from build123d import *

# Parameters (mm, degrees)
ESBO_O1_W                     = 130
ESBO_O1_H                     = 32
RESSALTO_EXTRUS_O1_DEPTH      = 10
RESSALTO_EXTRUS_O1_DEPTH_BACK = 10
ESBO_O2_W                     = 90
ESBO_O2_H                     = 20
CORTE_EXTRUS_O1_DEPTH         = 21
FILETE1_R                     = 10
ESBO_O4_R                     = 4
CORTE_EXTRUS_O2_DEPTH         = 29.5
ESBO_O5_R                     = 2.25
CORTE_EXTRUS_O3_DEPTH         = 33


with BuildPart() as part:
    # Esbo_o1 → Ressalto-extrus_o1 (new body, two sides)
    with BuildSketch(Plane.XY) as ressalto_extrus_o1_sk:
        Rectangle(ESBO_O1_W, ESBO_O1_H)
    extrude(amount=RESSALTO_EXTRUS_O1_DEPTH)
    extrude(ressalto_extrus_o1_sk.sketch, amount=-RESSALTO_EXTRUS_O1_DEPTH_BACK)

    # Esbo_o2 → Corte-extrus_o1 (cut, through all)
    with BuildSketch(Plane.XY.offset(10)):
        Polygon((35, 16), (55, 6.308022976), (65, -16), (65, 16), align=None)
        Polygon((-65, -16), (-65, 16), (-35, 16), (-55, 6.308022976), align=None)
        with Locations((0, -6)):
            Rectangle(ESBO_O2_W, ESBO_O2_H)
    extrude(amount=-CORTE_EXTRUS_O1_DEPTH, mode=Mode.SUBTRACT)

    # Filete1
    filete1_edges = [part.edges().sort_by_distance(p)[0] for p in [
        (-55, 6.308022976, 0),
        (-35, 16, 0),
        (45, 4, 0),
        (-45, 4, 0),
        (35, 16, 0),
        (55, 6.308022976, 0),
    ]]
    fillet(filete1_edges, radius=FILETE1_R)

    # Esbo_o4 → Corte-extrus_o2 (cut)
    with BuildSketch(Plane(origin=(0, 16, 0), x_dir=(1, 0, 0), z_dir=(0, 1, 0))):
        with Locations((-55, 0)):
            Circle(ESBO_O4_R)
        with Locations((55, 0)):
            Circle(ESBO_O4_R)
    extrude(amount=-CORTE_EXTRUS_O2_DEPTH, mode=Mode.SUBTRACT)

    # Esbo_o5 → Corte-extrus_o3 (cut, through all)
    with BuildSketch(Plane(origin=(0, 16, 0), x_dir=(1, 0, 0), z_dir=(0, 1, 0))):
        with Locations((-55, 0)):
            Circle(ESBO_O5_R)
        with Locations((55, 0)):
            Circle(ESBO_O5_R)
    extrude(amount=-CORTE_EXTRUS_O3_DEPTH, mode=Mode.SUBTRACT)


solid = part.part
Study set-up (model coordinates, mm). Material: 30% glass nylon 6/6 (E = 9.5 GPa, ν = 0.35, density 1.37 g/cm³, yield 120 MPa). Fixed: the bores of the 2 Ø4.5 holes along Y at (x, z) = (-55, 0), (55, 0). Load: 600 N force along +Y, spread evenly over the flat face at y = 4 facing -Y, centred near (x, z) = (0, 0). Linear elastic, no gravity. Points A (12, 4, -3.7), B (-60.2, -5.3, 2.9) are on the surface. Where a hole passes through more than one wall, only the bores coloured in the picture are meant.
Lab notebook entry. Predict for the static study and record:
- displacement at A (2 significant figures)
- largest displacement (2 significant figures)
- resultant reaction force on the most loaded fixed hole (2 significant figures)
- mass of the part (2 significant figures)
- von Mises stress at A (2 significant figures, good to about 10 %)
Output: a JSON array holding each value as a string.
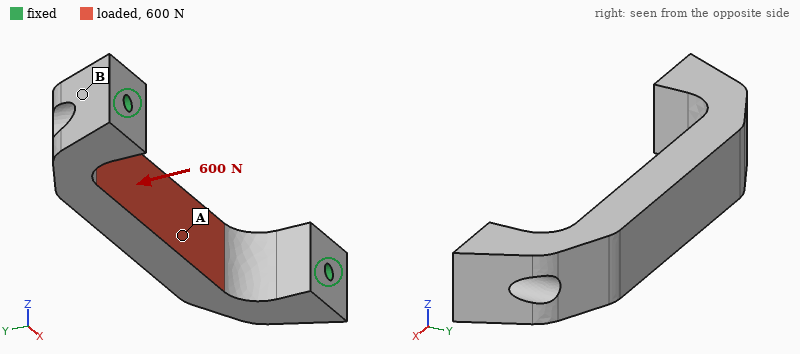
["0.10 mm", "0.11 mm", "420 N", "46 g", "5.4 MPa"]
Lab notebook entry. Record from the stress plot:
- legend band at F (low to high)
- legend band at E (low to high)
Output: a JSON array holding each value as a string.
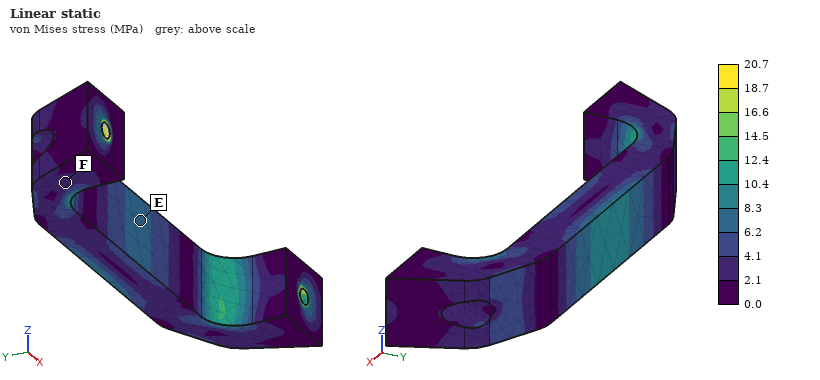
["2.1 to 4.1 MPa", "6.2 to 8.3 MPa"]
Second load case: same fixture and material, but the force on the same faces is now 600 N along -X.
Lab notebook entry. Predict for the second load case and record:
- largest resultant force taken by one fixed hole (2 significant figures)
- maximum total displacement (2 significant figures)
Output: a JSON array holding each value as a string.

["310 N", "0.13 mm"]
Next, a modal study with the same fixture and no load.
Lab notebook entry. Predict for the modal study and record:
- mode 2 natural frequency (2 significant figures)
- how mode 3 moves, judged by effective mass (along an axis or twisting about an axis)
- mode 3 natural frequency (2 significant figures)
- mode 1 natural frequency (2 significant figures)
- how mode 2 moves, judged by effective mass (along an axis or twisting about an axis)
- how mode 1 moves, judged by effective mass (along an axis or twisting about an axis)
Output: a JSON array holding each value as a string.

["1900 Hz", "twisting about Y", "2400 Hz", "780 Hz", "along X", "along Z"]
